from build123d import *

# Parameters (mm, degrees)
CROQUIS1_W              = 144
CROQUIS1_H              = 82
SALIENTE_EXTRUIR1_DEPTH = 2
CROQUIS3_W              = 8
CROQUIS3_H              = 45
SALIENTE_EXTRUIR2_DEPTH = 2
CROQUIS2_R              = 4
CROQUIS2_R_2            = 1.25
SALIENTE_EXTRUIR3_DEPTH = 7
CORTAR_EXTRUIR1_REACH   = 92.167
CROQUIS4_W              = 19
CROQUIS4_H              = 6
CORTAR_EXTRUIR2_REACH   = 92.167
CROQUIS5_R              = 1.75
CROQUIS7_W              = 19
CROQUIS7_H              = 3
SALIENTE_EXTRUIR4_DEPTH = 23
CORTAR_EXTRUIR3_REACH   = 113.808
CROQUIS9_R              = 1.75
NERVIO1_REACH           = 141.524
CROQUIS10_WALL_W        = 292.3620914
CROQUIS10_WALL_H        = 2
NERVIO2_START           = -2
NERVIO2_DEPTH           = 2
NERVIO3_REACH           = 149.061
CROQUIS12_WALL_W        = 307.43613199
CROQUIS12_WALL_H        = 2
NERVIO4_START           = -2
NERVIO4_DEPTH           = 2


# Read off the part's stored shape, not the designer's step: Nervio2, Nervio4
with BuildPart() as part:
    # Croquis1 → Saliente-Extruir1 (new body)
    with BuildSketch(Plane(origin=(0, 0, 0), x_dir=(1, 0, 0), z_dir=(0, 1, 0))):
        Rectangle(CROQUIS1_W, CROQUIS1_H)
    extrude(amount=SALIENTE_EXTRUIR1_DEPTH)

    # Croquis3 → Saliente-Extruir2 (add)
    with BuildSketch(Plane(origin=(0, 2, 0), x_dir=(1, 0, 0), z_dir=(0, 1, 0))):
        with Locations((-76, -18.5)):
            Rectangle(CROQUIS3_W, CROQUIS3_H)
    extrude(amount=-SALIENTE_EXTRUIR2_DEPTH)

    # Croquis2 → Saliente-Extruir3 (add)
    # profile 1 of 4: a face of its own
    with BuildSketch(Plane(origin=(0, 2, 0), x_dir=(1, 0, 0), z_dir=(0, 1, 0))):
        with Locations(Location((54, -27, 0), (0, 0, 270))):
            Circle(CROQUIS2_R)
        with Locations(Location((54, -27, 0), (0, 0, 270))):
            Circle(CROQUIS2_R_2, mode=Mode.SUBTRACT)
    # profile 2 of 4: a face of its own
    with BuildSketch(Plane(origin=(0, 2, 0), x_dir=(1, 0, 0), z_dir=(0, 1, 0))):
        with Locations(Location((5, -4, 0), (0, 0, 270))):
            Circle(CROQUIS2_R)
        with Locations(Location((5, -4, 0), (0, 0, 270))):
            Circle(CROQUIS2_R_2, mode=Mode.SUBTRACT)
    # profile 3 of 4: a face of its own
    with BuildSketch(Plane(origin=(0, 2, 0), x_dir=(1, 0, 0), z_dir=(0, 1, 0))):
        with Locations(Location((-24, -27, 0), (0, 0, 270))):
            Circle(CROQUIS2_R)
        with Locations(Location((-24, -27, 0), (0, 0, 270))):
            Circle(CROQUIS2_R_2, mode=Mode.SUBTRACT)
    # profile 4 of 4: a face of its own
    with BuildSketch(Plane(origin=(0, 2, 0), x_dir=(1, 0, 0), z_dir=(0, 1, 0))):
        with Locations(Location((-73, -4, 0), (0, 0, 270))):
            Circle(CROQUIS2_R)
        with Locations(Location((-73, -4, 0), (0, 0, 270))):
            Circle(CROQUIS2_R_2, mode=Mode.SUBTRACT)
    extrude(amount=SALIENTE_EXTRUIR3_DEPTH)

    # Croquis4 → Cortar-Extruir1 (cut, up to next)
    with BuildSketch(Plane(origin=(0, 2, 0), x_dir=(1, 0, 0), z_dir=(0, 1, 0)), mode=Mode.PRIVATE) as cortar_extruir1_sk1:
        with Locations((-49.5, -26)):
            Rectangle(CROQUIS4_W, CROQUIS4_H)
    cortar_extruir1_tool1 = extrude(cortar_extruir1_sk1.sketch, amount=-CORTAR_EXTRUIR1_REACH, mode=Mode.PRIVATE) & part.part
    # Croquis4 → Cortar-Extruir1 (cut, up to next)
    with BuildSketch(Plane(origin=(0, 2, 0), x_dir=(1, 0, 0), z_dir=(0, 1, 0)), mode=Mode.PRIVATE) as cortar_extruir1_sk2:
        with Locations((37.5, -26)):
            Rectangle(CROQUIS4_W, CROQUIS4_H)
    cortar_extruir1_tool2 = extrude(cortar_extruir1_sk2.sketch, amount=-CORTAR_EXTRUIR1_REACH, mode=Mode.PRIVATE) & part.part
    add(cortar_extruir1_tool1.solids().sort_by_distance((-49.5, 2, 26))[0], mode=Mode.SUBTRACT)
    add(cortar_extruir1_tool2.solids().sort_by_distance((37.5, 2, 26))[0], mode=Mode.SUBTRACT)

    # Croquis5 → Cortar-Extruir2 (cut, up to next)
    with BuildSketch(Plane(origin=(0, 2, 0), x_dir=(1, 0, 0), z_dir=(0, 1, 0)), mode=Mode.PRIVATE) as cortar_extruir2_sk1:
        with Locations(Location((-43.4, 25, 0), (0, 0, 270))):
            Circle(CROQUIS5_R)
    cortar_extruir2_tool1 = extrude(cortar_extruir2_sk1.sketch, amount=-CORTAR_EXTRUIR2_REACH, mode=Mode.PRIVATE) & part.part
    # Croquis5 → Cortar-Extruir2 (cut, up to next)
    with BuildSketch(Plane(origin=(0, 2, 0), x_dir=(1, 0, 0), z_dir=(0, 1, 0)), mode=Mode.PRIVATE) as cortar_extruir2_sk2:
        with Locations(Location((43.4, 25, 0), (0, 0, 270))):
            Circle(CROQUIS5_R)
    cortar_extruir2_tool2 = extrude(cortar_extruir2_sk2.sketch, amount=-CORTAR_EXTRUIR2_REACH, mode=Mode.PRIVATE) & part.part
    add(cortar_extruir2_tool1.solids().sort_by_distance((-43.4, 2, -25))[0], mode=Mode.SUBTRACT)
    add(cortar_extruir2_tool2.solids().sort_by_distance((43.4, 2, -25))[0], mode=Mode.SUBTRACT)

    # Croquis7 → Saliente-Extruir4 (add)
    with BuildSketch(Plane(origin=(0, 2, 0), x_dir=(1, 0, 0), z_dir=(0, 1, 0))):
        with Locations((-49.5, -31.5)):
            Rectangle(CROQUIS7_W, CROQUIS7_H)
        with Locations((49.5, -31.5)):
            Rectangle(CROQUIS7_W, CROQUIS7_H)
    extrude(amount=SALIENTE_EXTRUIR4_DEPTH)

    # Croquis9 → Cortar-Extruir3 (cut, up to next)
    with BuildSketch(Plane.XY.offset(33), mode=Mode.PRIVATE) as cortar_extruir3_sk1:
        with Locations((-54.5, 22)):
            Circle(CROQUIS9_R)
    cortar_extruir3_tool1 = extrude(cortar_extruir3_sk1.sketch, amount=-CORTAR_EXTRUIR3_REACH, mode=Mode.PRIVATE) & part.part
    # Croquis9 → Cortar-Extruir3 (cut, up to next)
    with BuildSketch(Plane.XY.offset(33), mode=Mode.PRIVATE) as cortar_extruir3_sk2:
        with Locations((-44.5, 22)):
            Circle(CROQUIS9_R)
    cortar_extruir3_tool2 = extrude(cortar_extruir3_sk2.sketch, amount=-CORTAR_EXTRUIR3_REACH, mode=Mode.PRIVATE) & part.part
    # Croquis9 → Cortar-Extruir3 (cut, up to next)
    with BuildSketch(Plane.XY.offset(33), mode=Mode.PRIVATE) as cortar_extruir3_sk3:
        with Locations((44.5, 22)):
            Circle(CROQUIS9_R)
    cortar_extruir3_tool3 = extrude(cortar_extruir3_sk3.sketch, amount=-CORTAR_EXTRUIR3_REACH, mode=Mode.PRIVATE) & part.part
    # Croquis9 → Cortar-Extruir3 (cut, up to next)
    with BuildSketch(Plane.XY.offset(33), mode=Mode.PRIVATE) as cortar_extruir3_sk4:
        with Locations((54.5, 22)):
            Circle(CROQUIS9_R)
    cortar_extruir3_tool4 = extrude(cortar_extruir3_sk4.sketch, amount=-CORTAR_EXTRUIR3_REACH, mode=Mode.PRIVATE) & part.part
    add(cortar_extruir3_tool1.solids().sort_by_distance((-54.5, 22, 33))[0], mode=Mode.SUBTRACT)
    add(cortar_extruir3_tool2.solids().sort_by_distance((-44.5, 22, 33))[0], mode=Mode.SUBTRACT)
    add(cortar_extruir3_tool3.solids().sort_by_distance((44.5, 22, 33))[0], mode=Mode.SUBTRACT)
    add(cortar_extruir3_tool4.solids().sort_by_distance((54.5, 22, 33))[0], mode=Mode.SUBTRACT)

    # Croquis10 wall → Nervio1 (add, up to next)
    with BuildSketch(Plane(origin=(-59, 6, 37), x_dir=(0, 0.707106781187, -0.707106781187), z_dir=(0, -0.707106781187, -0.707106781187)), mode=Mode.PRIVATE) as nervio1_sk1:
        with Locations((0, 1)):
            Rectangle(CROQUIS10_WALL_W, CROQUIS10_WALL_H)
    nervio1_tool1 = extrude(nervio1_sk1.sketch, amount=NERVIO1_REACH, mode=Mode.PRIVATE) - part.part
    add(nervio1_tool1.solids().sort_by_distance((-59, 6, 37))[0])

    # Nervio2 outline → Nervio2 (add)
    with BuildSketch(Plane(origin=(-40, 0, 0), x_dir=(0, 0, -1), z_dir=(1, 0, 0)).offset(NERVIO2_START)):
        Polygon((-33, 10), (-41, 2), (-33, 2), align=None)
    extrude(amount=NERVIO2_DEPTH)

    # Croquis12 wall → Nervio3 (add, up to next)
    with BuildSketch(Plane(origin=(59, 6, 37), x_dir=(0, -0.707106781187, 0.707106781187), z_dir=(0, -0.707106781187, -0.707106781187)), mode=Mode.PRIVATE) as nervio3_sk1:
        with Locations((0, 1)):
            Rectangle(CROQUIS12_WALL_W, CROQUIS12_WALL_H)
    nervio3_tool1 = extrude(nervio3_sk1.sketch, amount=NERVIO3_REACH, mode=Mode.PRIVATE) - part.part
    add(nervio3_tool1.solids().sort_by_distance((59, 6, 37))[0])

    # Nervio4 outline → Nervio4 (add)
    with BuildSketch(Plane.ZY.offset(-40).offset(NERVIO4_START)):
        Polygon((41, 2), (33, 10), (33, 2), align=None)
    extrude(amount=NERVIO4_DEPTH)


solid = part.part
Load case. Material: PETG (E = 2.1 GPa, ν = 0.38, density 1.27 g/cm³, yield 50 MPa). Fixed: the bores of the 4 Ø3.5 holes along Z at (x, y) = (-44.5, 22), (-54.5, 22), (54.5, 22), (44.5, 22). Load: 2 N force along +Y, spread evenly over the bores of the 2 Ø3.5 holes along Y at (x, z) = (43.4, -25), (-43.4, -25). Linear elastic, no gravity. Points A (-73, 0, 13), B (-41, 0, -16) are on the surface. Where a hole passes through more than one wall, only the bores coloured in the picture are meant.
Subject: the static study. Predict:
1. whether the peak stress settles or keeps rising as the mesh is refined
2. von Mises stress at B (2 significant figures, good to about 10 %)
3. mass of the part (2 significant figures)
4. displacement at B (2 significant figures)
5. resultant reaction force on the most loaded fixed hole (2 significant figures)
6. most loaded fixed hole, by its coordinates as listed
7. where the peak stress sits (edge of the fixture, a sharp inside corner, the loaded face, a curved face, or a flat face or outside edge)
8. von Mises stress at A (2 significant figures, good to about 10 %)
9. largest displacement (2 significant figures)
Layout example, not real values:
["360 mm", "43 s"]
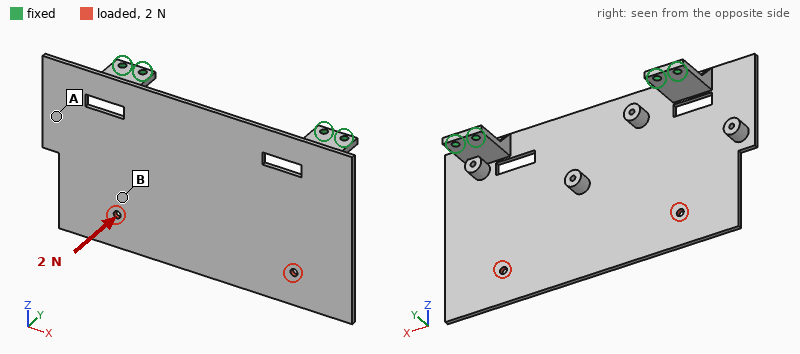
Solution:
["keeps rising", "0.32 MPa", "35 g", "1.2 mm", "1.00 N", "(54.5, 22)", "a sharp inside corner", "0.84 MPa", "2.0 mm"]
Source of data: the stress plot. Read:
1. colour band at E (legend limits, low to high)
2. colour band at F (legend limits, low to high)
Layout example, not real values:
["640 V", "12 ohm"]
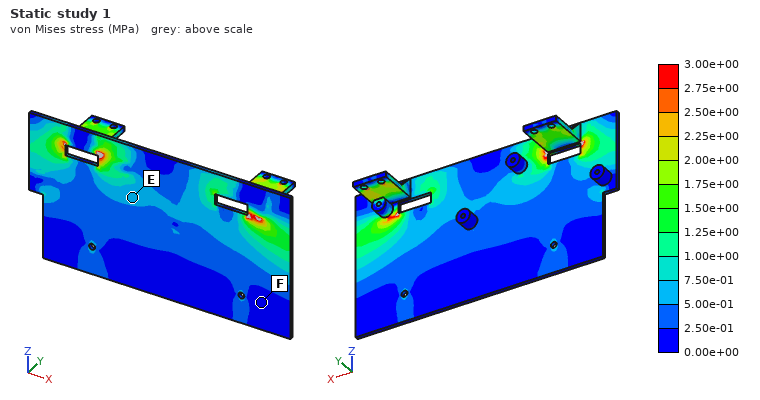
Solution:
["5.00e-01 to 7.50e-01 MPa", "0.00e+00 to 2.50e-01 MPa"]
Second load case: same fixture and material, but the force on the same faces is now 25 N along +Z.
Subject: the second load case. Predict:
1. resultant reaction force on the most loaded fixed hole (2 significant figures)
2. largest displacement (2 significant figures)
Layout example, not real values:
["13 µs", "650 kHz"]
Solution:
["6.4 N", "1.8 mm"]
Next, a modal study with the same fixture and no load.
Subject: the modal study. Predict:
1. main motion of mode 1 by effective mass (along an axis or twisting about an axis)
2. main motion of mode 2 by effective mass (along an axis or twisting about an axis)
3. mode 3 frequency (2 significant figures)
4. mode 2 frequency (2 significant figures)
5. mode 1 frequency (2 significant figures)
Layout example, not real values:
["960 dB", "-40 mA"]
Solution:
["along Y", "twisting about Z", "200 Hz", "100 Hz", "50 Hz"]
